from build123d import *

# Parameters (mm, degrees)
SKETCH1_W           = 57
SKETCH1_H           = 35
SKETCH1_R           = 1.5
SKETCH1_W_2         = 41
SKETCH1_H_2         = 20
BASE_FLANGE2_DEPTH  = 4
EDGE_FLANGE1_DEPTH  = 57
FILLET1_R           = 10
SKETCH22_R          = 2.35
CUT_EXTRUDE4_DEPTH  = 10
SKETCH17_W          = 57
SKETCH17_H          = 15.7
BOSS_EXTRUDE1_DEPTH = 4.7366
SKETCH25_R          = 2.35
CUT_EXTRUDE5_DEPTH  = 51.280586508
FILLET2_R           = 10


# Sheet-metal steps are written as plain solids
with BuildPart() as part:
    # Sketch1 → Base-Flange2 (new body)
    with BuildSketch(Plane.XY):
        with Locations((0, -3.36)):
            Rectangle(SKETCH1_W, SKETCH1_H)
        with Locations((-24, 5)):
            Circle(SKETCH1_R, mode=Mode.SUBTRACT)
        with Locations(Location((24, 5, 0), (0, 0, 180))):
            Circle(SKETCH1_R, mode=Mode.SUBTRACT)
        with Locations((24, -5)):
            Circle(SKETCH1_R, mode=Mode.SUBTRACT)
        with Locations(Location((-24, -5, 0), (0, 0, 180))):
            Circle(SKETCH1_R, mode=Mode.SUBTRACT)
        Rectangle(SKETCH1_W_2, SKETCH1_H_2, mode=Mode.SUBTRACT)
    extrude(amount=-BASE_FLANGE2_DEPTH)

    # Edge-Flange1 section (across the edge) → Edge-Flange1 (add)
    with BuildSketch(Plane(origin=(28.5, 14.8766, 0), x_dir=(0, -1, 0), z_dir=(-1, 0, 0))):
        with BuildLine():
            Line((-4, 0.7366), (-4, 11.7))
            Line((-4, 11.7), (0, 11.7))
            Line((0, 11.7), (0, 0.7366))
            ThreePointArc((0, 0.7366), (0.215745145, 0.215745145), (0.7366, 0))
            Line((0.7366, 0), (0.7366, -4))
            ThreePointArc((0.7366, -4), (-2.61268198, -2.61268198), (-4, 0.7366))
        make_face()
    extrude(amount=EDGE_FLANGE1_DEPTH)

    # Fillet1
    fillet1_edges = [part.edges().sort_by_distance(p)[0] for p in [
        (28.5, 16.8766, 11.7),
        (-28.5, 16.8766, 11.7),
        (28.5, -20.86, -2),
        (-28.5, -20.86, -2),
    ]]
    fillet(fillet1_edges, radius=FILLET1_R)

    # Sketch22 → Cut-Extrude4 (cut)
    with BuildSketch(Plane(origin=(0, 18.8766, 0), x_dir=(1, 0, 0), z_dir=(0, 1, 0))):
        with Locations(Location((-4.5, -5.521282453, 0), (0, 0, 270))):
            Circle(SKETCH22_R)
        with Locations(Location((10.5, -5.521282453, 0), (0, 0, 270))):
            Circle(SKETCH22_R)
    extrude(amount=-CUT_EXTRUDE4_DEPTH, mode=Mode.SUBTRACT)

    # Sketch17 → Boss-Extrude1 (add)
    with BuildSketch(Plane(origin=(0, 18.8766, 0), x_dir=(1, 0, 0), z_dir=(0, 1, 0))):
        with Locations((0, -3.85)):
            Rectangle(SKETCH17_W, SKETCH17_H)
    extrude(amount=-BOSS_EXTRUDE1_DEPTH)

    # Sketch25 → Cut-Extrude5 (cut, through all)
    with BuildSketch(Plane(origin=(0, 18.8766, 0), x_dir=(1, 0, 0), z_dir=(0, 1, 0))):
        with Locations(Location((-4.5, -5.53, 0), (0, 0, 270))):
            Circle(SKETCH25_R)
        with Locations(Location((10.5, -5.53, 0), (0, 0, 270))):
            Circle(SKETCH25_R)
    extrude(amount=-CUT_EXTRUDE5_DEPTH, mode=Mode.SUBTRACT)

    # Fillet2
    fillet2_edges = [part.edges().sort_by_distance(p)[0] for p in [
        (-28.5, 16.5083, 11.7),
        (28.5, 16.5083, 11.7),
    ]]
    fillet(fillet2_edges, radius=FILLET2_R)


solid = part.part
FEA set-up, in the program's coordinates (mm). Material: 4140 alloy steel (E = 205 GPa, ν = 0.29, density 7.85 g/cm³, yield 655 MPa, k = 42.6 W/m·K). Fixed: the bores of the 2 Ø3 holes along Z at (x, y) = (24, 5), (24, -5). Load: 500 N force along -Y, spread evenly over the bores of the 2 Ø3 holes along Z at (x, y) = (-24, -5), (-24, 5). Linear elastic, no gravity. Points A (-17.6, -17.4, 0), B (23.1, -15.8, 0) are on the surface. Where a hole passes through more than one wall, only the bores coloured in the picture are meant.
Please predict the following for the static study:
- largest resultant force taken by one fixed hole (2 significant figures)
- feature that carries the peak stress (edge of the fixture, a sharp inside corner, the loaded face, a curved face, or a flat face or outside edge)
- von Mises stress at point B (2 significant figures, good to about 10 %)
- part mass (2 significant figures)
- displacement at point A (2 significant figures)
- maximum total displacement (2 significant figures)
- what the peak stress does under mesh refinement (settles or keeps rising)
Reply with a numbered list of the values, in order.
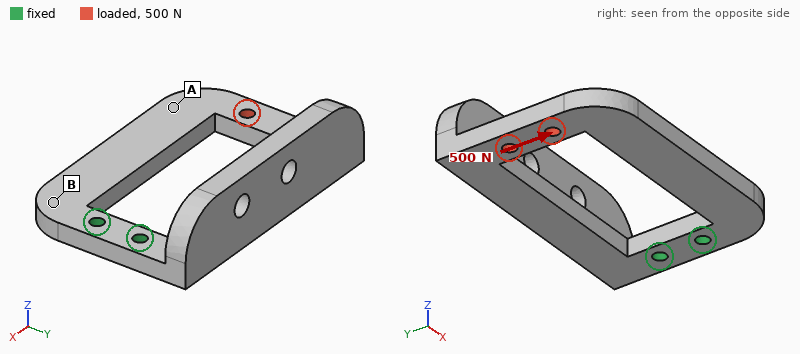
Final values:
1. 1.2 kN
2. edge of the fixture
3. 61 MPa
4. 65 g
5. 0.13 mm
6. 0.16 mm
7. keeps rising
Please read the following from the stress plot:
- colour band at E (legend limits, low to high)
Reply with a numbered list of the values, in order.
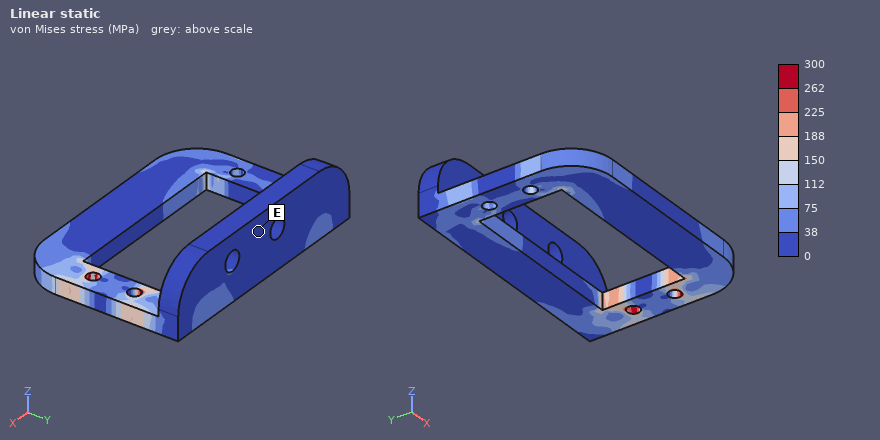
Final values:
1. 0 to 38 MPa
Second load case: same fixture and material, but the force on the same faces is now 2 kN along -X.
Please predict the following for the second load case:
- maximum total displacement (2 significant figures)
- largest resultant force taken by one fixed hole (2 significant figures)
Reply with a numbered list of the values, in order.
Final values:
1. 34 µm
2. 1.0 kN
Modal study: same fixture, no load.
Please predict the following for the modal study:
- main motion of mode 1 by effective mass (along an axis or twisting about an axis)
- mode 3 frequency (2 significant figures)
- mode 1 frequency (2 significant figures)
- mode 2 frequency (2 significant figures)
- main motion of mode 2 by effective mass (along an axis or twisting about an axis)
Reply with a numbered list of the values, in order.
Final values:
1. along Z
2. 2000 Hz
3. 870 Hz
4. 1700 Hz
5. along Y
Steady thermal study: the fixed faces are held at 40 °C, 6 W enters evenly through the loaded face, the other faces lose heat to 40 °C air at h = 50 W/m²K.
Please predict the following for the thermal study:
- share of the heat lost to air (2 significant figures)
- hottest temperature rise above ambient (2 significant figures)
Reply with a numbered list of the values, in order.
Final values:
1. 73 %
2. 50 K
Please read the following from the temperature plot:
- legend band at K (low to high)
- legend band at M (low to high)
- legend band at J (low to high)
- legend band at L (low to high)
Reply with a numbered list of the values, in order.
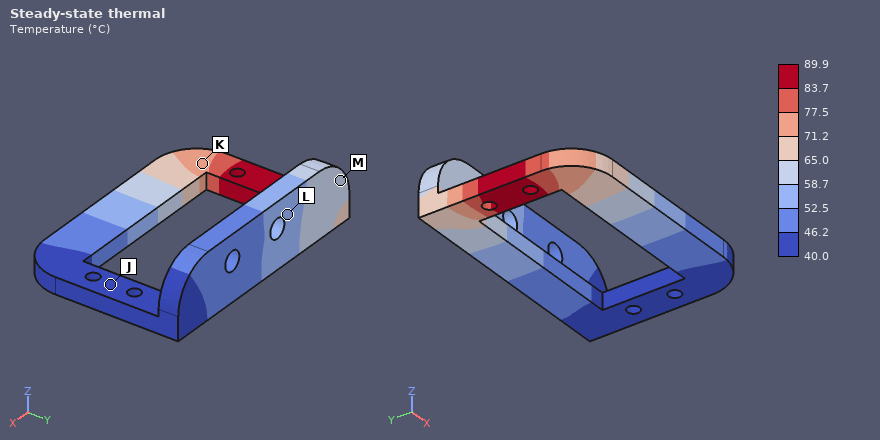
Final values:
1. 71.2 to 77.5 °C
2. 58.7 to 65.0 °C
3. 40.0 to 46.2 °C
4. 52.5 to 58.7 °C
